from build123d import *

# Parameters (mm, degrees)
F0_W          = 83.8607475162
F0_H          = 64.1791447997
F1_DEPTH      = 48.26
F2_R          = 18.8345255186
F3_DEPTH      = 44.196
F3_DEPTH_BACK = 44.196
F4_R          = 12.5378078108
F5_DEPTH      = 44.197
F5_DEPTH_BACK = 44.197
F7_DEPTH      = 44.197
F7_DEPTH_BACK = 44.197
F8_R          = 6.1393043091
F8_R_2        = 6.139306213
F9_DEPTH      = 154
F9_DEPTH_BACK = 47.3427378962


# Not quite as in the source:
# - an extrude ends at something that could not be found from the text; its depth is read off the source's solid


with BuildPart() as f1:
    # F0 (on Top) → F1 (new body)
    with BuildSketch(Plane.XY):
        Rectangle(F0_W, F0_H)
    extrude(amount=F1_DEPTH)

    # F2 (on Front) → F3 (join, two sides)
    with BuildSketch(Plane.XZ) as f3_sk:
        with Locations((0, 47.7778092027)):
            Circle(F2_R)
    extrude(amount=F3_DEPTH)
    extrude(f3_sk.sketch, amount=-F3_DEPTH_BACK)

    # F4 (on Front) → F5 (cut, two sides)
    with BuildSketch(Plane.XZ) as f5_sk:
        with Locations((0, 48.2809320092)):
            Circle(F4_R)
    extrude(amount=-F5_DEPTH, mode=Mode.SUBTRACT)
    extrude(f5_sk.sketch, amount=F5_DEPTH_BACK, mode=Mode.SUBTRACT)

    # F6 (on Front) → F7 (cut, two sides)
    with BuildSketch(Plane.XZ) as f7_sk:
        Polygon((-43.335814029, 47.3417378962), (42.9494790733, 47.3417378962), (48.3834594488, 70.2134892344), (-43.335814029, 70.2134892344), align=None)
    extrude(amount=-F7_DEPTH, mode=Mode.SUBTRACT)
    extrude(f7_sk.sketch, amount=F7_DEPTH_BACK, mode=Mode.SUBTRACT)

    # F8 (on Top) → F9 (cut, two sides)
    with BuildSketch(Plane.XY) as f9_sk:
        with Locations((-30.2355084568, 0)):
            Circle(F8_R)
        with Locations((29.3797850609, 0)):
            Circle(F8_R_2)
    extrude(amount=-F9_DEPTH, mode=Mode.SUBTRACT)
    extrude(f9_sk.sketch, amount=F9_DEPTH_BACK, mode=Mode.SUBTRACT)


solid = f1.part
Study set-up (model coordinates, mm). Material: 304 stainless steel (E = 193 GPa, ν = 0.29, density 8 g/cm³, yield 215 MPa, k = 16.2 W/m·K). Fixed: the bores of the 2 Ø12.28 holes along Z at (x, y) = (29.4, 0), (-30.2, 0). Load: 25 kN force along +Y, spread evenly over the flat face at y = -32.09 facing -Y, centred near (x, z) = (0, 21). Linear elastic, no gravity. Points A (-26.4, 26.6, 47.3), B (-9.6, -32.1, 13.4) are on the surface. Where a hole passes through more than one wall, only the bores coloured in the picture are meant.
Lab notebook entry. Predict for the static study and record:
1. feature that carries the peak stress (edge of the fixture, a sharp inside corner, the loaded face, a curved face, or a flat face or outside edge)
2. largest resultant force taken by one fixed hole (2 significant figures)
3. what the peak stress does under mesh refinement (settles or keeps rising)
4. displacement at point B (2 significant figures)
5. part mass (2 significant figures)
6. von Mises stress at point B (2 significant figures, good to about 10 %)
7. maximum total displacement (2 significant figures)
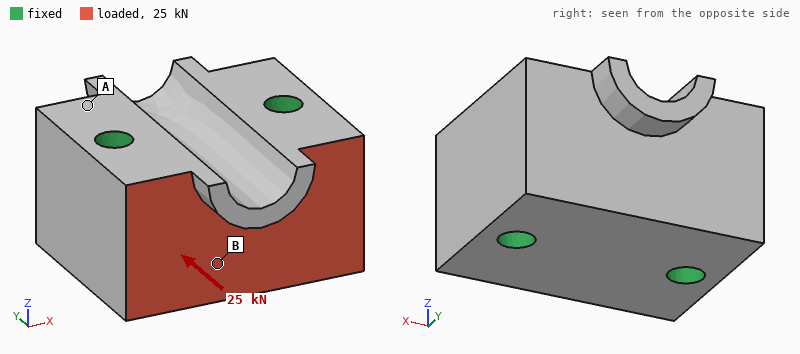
edge of the fixture
13 kN
keeps rising
1.6 µm
1.9 kg
5.8 MPa
1.9 µm
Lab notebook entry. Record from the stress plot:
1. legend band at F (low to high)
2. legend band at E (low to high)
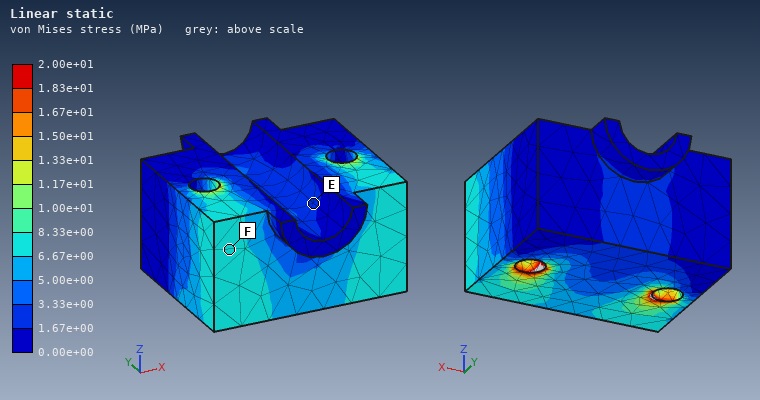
6.67e+00 to 8.33e+00 MPa
1.67e+00 to 3.33e+00 MPa
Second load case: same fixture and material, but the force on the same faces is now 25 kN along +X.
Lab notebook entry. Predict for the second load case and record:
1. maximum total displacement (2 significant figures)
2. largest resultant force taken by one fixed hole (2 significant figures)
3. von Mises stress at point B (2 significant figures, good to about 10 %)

5.9 µm
17 kN
13 MPa
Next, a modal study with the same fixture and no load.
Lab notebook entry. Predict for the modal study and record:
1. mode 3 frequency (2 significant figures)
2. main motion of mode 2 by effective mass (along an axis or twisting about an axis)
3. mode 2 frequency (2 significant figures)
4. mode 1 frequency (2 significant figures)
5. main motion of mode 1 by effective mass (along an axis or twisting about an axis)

19 kHz
along Z
16 kHz
15 kHz
twisting about X
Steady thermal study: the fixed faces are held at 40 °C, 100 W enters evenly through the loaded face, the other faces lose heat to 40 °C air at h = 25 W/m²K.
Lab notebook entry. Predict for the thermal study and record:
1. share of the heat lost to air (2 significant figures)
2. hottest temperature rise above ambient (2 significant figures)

8.0 %
55 K
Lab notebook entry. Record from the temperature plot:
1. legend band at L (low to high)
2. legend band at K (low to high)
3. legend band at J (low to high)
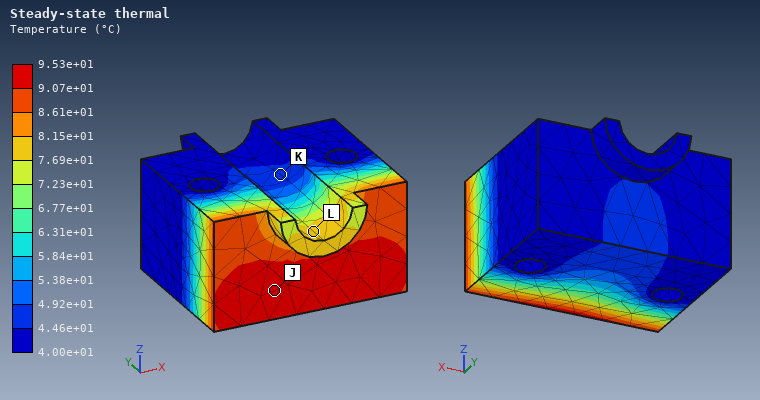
7.69e+01 to 8.15e+01 °C
4.46e+01 to 4.92e+01 °C
9.07e+01 to 9.53e+01 °C
